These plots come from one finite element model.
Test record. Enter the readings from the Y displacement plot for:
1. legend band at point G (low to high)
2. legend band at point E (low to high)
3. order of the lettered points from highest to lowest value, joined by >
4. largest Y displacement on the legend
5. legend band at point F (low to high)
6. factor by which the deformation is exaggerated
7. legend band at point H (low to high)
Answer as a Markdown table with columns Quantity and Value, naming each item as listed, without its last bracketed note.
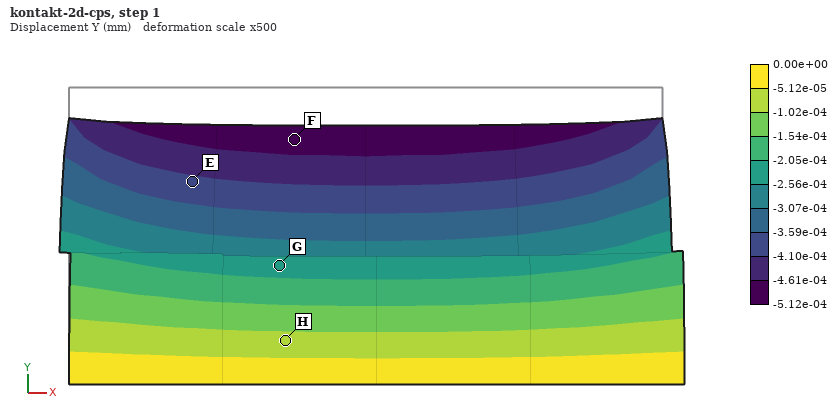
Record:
| Quantity | Value |
|---|---|
| legend band at point G | -2.56e-04 to -2.05e-04 mm |
| legend band at point E | -4.10e-04 to -3.59e-04 mm |
| order of the lettered points from highest to lowest value, joined by > | H > G > E > F |
| largest Y displacement on the legend | 0.00e+00 mm |
| legend band at point F | -5.12e-04 to -4.61e-04 mm |
| factor by which the deformation is exaggerated | 500 |
| legend band at point H | -1.02e-04 to -5.12e-05 mm |
